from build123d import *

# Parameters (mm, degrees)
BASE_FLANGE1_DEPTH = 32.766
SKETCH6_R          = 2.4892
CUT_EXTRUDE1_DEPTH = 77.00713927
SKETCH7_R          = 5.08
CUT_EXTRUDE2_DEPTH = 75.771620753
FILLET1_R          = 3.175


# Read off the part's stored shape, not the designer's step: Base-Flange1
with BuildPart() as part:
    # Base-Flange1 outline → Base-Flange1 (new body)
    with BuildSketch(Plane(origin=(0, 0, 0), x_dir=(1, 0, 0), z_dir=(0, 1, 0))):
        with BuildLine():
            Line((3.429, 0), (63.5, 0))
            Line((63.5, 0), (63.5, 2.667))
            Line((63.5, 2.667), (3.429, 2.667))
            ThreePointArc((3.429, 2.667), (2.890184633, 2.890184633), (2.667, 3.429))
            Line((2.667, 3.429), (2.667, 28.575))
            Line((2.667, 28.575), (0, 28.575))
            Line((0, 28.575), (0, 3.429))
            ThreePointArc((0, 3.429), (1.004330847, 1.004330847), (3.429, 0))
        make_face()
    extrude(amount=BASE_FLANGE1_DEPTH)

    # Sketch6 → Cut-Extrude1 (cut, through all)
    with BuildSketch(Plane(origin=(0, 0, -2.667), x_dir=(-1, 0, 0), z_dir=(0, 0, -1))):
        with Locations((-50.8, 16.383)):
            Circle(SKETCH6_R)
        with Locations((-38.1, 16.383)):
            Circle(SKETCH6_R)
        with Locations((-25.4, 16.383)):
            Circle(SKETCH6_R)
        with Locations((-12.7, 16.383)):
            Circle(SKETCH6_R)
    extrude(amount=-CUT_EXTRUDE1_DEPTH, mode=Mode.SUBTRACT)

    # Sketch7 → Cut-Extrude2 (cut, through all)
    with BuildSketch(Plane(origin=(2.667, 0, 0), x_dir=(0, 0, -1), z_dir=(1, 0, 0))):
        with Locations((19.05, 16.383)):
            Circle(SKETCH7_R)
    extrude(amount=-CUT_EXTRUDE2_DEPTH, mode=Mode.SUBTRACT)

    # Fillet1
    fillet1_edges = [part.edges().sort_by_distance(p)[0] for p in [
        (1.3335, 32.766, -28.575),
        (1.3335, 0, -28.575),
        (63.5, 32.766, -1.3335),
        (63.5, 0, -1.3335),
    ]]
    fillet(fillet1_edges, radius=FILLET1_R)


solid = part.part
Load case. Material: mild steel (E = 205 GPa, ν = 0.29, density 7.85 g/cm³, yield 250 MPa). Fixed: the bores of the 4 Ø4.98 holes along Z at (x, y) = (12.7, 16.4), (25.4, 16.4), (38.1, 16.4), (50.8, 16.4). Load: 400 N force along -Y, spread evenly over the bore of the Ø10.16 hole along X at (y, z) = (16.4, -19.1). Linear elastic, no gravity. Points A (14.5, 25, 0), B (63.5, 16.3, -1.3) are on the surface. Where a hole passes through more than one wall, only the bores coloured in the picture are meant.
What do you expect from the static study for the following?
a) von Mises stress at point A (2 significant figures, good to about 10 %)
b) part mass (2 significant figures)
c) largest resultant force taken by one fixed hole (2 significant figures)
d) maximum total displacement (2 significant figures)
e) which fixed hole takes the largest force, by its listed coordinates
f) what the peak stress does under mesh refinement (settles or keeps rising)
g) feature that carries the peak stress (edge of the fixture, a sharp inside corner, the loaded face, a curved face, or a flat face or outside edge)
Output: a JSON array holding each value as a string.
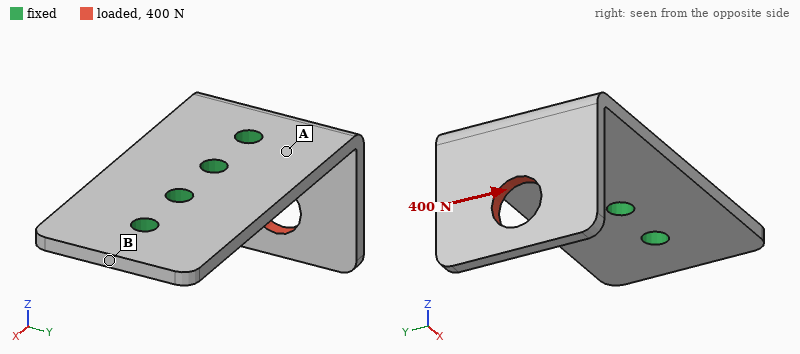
["85 MPa", "57 g", "520 N", "0.12 mm", "(12.7, 16.4)", "keeps rising", "edge of the fixture"]
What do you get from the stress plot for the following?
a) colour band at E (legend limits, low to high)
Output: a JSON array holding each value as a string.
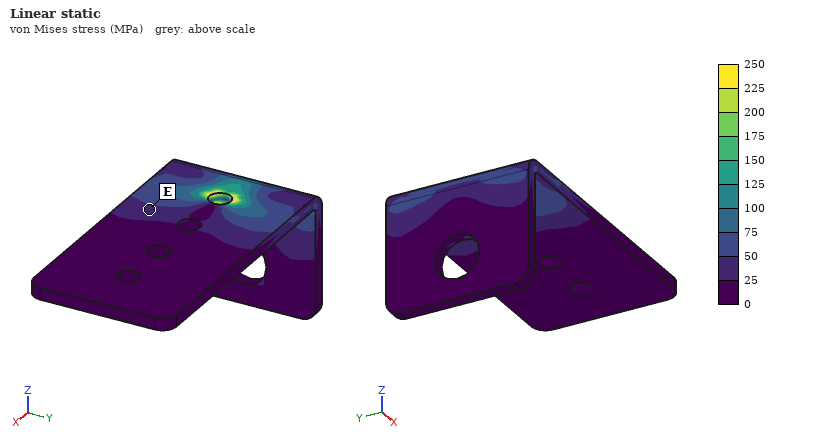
["25 to 50 MPa"]
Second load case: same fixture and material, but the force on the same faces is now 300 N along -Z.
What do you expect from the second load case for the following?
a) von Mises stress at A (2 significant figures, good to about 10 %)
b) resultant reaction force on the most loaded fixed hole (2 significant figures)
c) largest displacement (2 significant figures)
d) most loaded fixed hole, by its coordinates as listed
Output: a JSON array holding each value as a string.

["26 MPa", "370 N", "52 µm", "(12.7, 16.4)"]
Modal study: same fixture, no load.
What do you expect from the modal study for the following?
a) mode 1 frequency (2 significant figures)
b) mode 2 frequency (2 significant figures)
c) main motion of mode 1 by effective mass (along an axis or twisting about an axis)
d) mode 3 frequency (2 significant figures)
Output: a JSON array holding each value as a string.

["1900 Hz", "2700 Hz", "along X", "5400 Hz"]
